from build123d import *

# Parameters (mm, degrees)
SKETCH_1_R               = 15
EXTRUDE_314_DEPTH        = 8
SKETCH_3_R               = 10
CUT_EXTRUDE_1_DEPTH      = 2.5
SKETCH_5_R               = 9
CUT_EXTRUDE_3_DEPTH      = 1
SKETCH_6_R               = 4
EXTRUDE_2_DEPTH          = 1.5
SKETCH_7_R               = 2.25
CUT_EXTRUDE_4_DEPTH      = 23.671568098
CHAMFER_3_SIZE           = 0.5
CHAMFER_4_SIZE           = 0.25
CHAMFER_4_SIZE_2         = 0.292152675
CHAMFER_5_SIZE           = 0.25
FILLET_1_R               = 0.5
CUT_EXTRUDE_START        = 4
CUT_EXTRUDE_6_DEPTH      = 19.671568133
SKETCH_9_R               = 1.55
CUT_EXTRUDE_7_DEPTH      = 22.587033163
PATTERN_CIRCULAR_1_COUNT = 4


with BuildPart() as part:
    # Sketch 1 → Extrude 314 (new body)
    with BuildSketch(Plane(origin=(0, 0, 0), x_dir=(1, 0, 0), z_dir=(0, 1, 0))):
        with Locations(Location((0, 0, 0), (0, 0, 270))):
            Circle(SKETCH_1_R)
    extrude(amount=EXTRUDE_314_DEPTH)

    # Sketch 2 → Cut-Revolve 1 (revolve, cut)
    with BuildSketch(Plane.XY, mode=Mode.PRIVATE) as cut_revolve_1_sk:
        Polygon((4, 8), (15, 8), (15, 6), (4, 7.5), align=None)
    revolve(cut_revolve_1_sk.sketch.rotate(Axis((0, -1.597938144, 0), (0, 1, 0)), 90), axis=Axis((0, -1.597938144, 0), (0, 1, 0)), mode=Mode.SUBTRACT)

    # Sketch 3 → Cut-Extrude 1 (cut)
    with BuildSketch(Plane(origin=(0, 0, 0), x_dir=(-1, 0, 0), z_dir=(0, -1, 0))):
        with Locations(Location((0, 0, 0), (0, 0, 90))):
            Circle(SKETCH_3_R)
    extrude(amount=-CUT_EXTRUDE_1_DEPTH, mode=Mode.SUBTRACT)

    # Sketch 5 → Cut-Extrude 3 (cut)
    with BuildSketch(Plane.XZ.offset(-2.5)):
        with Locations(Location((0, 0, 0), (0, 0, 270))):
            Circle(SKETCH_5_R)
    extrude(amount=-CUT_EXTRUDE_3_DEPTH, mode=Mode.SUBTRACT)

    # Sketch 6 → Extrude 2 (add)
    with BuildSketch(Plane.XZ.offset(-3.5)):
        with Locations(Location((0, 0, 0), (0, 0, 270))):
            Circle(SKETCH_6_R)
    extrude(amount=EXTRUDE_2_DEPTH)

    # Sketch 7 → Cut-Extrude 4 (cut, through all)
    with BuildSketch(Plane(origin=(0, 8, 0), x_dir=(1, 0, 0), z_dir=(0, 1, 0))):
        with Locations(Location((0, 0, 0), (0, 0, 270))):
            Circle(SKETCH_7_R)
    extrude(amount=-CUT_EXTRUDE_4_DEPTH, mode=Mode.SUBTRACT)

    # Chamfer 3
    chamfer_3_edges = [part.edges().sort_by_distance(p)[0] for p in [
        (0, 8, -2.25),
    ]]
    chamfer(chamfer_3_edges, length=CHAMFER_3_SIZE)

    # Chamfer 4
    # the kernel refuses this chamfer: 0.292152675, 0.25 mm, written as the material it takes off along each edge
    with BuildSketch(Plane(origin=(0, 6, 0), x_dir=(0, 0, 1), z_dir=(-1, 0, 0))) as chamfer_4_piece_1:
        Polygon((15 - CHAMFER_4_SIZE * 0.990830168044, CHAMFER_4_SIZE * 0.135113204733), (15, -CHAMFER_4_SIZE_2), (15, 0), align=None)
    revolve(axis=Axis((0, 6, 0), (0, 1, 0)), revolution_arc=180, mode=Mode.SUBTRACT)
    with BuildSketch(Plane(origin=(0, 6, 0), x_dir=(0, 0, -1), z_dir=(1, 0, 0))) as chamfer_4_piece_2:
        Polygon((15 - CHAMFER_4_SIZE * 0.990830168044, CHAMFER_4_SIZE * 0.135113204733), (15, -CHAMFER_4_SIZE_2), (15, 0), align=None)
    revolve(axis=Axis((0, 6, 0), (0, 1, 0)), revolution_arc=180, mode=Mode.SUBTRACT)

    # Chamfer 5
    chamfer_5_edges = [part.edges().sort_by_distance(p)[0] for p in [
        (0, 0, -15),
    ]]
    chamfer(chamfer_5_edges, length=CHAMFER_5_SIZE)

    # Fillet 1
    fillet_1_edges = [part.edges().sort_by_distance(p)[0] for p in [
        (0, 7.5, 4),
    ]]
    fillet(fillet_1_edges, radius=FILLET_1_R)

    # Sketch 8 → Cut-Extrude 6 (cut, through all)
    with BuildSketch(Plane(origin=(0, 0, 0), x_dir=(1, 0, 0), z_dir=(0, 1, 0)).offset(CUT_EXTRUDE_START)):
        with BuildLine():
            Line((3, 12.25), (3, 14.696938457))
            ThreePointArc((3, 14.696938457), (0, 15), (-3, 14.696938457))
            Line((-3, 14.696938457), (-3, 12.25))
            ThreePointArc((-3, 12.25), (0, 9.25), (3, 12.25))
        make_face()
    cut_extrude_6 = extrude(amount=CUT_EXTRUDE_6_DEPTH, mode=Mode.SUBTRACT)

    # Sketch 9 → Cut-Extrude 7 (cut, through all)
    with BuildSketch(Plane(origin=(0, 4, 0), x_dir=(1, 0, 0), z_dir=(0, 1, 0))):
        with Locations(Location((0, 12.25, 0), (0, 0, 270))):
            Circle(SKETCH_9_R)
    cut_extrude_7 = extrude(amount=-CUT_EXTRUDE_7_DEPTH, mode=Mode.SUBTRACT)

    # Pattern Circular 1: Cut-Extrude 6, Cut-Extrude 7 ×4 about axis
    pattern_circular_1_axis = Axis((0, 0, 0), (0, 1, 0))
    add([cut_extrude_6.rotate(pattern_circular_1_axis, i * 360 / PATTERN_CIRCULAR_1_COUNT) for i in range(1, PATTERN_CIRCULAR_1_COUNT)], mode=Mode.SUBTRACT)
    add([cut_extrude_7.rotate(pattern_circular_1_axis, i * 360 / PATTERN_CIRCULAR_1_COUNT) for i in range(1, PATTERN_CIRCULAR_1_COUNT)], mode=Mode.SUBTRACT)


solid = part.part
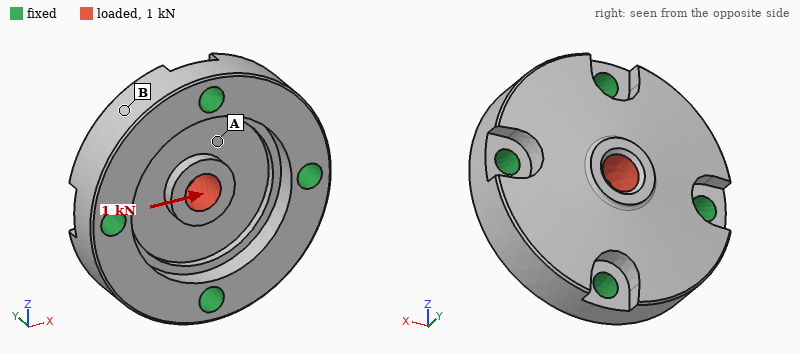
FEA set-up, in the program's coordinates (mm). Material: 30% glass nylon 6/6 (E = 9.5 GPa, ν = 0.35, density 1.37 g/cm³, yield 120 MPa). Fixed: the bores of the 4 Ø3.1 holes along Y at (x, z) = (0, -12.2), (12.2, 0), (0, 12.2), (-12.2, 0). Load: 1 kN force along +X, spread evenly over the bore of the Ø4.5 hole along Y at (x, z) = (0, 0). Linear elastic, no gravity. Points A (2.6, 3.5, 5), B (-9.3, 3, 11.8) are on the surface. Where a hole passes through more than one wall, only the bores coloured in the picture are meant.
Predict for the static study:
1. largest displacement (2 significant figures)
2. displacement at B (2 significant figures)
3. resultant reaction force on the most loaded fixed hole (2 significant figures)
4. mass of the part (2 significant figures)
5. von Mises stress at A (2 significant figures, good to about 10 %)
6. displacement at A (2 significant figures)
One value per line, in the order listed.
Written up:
32 µm
8.5 µm
280 N
4.5 g
14 MPa
15 µm
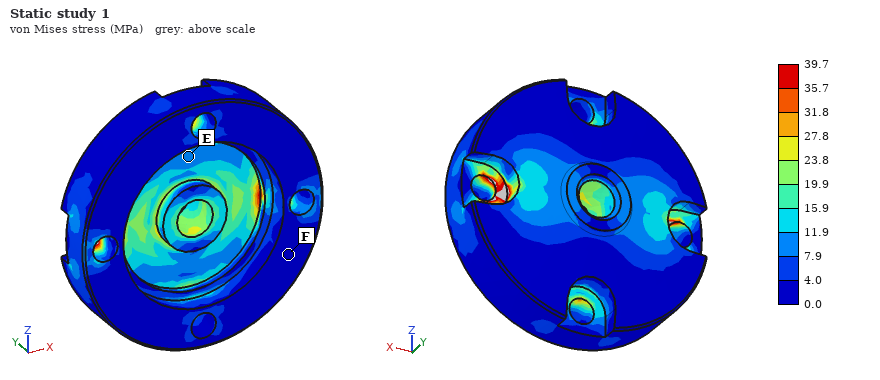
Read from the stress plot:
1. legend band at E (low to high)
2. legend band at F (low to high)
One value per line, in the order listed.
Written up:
7.9 to 11.9 MPa
0.0 to 4.0 MPa
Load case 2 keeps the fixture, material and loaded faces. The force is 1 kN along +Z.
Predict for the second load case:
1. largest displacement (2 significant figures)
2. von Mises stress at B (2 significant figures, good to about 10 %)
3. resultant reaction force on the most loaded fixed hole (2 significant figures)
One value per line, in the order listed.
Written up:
32 µm
3.5 MPa
280 N
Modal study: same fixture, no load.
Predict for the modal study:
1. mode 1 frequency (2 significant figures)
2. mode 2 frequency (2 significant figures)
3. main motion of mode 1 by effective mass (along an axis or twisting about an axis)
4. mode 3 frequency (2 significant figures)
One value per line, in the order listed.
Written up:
24 kHz
25 kHz
along Y
25 kHz
